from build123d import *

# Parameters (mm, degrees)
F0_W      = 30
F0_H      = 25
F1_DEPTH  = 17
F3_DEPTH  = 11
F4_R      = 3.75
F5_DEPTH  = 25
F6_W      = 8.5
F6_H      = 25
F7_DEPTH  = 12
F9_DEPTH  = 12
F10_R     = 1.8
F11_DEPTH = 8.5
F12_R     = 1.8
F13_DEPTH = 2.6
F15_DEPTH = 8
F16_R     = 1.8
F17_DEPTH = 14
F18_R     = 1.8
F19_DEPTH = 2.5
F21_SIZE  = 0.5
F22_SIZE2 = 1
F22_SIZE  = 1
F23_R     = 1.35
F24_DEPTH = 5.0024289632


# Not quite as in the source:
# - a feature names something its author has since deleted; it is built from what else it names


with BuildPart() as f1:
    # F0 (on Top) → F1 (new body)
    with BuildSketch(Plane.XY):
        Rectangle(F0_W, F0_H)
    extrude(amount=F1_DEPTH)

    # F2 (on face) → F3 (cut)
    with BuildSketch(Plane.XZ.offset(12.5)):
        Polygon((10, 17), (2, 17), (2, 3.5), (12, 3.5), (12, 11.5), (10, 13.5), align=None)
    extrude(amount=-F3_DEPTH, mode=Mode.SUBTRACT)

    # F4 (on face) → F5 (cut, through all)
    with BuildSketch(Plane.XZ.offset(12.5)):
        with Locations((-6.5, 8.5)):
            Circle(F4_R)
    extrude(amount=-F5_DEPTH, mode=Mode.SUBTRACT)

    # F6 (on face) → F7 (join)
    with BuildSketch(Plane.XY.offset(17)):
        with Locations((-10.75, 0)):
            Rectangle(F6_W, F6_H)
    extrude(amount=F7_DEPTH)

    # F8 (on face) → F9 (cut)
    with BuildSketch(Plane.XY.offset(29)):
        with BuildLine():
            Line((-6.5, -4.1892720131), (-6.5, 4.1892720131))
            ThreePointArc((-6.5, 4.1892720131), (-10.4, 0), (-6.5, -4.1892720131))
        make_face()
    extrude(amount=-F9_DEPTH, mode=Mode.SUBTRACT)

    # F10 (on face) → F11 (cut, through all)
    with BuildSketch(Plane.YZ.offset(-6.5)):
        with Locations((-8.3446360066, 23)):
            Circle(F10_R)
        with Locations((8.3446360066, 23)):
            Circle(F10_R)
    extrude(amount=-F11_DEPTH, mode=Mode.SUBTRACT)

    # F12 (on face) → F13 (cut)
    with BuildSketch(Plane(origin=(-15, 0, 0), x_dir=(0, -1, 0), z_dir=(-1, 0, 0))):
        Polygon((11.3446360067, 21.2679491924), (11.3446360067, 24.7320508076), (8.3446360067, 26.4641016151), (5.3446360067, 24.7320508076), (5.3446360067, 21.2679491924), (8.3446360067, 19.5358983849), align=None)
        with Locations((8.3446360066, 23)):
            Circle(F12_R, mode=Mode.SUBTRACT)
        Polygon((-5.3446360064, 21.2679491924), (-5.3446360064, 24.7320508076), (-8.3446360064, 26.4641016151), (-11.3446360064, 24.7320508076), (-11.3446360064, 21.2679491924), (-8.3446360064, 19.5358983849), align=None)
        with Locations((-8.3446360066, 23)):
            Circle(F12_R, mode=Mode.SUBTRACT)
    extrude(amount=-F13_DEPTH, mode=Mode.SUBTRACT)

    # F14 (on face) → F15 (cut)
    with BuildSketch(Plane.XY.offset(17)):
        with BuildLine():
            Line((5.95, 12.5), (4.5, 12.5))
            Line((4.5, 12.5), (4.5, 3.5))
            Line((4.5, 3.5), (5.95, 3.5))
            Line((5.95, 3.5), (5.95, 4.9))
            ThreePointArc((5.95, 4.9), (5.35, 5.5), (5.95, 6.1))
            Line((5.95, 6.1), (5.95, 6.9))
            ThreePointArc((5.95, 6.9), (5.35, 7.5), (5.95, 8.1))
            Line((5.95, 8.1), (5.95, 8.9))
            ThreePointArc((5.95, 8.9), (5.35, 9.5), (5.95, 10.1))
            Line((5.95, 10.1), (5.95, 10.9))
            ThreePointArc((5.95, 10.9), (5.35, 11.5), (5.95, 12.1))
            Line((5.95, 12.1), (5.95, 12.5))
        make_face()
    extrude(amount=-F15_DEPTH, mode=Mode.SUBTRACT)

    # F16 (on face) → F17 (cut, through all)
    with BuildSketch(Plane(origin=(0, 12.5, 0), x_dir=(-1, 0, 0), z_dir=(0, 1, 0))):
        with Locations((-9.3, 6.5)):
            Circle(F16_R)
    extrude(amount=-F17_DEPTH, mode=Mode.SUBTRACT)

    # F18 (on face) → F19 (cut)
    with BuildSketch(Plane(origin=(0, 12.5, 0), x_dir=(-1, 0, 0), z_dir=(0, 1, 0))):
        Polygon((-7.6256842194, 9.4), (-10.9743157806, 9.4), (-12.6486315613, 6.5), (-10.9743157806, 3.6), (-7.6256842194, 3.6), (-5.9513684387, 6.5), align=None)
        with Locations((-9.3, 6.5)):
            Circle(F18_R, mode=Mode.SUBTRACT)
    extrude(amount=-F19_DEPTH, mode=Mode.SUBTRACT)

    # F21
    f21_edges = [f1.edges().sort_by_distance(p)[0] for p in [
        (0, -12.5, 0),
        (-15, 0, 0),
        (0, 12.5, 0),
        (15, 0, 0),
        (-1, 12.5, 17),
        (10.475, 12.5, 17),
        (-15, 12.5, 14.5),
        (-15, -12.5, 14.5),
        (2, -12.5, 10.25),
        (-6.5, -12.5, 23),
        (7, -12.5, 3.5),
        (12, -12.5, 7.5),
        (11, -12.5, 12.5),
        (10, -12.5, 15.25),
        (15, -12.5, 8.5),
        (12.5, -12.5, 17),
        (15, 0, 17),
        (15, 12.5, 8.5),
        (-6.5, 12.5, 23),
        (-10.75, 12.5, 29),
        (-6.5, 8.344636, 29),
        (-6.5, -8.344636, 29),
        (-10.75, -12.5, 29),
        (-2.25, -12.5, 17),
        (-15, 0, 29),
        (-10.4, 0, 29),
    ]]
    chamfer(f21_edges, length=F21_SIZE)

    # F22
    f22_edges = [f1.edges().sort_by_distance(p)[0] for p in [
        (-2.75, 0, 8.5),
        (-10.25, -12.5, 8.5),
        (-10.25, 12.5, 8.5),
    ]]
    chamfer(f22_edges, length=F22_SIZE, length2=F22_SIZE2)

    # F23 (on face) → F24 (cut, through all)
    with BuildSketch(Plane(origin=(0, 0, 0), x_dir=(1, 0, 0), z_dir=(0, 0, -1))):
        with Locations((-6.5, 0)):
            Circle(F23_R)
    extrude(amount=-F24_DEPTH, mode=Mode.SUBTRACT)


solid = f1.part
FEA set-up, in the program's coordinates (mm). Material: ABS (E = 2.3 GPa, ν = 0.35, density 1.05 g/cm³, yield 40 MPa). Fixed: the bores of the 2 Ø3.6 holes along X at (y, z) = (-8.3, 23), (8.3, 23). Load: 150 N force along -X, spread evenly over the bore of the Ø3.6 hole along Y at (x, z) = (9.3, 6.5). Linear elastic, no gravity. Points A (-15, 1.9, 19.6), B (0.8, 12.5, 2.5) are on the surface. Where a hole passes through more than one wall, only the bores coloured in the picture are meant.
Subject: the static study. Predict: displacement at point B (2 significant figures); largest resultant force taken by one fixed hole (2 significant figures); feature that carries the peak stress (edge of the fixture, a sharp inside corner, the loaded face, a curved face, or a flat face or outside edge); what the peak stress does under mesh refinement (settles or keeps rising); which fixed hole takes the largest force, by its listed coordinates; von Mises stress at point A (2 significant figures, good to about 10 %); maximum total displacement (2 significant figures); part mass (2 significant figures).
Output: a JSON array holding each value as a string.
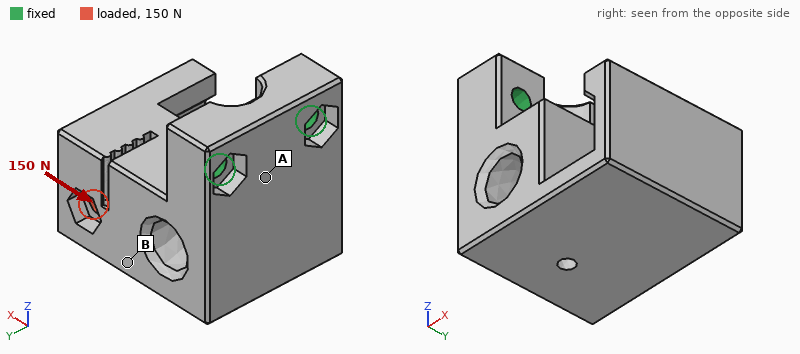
["0.27 mm", "110 N", "edge of the fixture", "keeps rising", "(8.3, 23)", "5.5 MPa", "0.40 mm", "12 g"]
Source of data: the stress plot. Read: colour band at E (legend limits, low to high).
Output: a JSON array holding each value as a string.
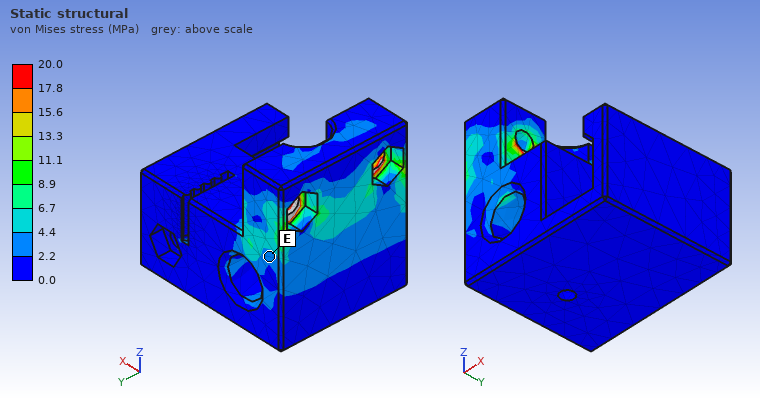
["2.2 to 4.4 MPa"]
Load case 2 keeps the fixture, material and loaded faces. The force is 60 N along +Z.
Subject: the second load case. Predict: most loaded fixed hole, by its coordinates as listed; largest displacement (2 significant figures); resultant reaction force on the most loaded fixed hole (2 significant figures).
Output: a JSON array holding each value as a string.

["(8.3, 23)", "0.25 mm", "45 N"]
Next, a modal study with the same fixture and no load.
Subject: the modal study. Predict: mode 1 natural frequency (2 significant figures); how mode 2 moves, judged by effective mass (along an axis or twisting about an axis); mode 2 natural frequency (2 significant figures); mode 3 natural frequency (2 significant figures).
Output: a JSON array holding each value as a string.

["1100 Hz", "along Y", "2100 Hz", "4300 Hz"]
